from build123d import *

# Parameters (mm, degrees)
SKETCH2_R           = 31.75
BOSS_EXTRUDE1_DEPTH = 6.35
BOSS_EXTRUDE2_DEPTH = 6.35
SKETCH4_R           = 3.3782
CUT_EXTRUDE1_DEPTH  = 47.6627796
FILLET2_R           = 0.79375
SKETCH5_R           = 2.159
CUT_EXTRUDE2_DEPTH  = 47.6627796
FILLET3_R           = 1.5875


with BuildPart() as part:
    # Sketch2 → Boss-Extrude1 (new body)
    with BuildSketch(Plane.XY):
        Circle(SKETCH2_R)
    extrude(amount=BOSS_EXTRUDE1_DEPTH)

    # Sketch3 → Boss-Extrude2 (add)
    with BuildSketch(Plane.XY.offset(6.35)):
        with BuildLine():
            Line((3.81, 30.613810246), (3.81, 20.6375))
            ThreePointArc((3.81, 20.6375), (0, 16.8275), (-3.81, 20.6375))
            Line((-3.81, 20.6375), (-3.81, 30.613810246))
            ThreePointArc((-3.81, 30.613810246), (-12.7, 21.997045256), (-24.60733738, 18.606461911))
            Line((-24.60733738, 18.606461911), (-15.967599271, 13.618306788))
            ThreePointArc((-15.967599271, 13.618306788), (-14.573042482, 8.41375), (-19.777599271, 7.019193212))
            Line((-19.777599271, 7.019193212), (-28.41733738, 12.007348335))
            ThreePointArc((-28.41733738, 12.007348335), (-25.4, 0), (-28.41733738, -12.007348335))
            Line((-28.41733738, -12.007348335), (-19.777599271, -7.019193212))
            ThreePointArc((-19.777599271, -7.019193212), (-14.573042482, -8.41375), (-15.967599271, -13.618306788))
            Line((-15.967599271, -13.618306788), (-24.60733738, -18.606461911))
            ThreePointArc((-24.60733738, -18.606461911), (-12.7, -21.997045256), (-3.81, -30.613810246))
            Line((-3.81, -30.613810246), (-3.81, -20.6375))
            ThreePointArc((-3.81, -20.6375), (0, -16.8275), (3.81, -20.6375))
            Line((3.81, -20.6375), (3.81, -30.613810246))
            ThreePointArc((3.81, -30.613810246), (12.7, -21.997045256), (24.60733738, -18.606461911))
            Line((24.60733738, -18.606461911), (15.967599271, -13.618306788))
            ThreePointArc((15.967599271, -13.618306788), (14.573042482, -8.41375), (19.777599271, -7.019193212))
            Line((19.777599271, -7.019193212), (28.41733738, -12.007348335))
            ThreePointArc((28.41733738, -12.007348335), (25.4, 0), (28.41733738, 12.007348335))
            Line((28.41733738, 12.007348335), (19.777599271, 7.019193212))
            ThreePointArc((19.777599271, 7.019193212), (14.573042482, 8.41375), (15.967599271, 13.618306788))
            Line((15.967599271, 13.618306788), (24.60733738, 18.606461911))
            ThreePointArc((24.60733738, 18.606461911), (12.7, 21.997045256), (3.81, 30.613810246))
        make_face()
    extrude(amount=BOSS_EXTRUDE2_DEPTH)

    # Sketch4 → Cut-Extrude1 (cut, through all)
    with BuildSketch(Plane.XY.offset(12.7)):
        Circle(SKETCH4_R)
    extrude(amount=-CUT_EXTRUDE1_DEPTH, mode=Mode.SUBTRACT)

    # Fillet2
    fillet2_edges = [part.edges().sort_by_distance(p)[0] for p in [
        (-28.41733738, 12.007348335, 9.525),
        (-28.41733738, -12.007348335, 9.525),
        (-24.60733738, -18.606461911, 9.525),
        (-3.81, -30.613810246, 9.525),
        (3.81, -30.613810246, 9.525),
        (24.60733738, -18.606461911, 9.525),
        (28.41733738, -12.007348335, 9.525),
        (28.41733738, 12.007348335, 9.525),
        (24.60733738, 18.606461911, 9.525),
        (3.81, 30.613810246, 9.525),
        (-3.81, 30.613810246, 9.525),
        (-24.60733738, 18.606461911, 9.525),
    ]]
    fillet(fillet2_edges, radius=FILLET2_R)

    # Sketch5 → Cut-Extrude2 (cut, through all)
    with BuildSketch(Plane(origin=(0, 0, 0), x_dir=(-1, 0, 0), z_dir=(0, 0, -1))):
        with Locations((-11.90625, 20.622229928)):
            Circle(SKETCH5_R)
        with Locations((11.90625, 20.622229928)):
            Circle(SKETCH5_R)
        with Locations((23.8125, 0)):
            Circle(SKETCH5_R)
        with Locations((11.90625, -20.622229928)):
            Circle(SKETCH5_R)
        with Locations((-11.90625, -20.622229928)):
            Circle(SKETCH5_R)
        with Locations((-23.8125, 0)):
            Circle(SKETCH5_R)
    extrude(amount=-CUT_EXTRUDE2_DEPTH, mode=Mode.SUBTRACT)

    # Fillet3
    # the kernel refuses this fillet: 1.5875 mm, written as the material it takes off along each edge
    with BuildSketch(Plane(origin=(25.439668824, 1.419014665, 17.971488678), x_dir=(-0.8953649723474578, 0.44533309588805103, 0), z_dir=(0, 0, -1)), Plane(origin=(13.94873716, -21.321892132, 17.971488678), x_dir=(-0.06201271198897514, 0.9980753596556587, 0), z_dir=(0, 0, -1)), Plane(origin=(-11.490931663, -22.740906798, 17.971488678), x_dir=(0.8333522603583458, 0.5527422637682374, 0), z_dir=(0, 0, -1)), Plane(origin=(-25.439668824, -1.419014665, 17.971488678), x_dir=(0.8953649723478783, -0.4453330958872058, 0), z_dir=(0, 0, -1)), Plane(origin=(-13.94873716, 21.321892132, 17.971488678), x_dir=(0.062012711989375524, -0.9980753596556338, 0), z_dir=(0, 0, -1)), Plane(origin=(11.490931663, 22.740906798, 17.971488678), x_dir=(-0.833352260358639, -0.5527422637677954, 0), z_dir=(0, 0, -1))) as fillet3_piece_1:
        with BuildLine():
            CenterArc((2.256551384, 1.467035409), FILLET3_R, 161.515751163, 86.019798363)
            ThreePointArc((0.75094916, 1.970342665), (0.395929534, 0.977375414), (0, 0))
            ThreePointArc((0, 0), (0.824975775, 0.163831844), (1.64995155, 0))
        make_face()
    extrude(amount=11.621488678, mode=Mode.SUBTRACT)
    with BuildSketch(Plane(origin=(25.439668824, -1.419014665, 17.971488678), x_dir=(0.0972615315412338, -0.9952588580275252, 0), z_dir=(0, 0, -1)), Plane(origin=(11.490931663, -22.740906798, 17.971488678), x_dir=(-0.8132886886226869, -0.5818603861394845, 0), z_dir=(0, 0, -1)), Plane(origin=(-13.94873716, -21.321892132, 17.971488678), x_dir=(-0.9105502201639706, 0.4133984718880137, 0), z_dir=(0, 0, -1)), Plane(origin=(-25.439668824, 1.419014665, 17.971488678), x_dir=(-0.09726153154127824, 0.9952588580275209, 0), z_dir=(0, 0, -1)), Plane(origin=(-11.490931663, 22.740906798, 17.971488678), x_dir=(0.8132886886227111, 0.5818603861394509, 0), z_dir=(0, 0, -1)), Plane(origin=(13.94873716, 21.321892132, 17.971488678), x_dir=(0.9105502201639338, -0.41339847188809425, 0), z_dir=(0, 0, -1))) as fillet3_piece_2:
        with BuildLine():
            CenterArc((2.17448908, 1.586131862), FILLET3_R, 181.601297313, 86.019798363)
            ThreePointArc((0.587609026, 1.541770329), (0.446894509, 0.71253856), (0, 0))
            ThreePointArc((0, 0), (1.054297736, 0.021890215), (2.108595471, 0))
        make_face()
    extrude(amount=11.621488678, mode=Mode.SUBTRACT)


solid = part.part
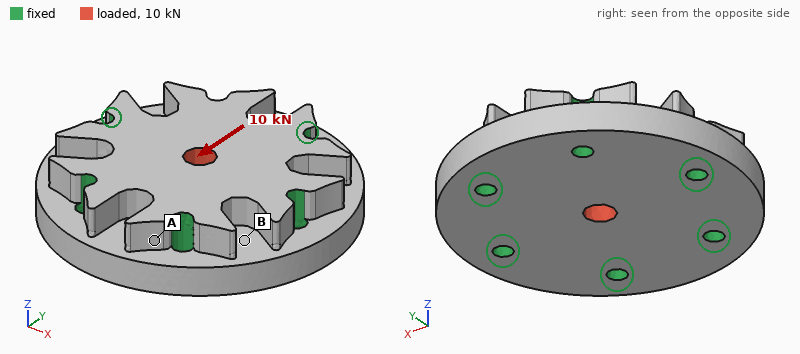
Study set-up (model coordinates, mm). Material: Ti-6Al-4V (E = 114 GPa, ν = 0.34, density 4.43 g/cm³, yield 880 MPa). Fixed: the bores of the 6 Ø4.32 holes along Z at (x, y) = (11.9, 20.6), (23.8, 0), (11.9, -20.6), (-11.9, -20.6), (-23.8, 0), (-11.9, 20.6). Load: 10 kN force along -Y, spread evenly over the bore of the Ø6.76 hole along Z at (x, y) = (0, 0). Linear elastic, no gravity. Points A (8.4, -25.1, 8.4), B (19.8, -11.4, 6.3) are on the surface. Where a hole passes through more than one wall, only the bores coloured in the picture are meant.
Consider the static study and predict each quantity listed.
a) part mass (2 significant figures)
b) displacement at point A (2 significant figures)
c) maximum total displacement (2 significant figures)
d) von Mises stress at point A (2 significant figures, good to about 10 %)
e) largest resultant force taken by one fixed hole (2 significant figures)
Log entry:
130 g
0.76 µm
4.2 µm
9.3 MPa
2.4 kN
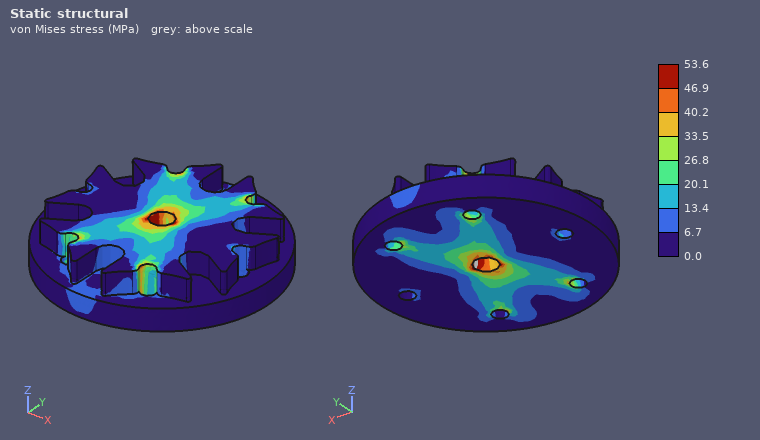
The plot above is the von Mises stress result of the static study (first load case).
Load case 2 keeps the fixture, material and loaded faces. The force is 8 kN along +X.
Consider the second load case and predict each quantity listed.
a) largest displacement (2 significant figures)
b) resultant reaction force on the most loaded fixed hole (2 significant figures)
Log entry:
3.4 µm
2.2 kN
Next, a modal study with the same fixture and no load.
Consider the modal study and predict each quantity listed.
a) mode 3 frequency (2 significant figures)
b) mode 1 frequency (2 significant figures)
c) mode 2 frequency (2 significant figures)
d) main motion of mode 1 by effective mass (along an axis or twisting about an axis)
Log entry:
44 kHz
31 kHz
44 kHz
along Z
